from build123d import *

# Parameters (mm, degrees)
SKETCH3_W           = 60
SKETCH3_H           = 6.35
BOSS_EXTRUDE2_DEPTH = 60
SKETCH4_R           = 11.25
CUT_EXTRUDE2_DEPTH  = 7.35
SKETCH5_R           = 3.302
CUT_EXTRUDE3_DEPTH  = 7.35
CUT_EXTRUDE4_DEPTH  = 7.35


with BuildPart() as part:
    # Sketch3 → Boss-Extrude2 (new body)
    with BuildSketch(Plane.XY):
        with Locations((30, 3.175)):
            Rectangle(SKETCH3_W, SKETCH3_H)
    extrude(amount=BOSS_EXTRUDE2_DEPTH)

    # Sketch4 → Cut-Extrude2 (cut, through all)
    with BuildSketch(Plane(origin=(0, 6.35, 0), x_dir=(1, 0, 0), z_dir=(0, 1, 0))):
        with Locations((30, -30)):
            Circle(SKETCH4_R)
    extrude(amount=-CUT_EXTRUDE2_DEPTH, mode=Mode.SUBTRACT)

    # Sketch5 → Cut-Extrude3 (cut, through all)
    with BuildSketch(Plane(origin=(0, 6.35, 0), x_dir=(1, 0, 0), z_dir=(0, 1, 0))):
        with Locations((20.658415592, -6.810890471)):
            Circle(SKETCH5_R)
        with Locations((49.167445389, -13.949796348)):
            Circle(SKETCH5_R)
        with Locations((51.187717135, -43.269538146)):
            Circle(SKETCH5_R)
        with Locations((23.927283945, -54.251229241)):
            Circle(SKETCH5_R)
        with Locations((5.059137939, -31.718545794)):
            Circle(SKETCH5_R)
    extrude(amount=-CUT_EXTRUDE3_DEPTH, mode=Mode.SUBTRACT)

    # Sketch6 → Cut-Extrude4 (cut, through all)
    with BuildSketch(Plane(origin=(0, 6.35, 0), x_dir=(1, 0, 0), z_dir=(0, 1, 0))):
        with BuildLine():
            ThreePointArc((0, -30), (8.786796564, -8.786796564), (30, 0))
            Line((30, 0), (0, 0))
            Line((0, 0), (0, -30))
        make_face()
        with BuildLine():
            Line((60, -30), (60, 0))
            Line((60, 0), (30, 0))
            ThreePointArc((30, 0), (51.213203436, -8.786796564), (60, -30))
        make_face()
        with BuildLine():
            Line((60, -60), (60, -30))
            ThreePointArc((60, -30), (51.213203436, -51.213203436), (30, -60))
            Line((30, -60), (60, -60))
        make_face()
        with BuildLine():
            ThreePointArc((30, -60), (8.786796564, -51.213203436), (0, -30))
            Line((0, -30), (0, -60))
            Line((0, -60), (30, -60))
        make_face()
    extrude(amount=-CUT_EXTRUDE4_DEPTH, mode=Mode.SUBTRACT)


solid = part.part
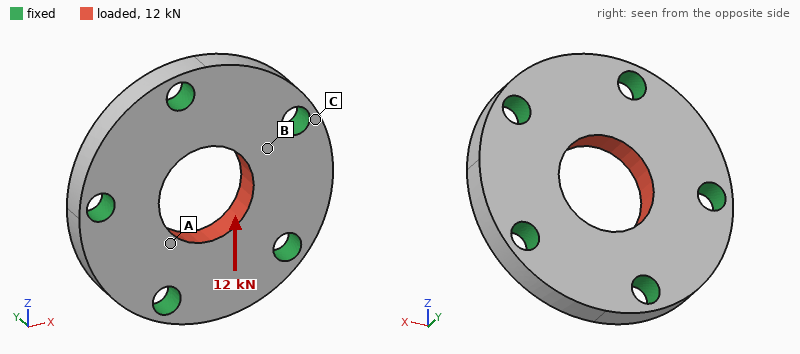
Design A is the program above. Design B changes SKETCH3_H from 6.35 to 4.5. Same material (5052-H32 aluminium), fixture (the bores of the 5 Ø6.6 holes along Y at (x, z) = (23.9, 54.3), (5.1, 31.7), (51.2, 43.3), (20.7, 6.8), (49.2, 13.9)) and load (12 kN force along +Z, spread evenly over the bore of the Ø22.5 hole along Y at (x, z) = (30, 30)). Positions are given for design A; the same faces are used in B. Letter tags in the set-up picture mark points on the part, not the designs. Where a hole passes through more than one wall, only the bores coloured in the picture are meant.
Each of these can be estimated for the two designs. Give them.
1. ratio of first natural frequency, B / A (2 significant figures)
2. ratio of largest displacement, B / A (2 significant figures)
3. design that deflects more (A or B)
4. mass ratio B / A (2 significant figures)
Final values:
0.81
1.4
B
0.71
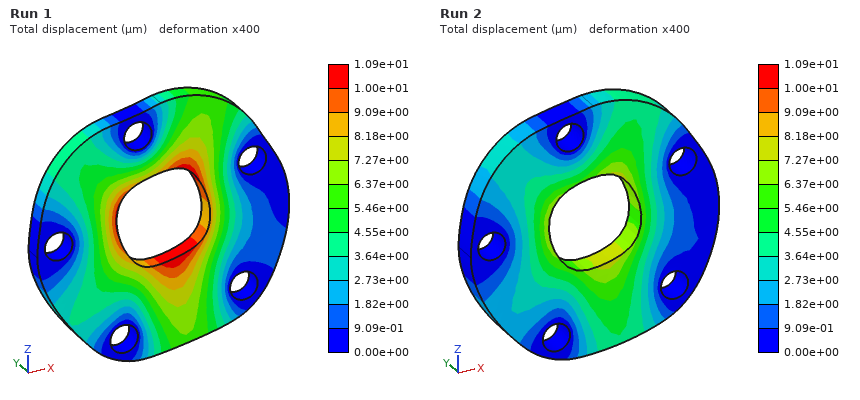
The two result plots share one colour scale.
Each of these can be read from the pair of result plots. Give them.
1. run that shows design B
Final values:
Run 1
